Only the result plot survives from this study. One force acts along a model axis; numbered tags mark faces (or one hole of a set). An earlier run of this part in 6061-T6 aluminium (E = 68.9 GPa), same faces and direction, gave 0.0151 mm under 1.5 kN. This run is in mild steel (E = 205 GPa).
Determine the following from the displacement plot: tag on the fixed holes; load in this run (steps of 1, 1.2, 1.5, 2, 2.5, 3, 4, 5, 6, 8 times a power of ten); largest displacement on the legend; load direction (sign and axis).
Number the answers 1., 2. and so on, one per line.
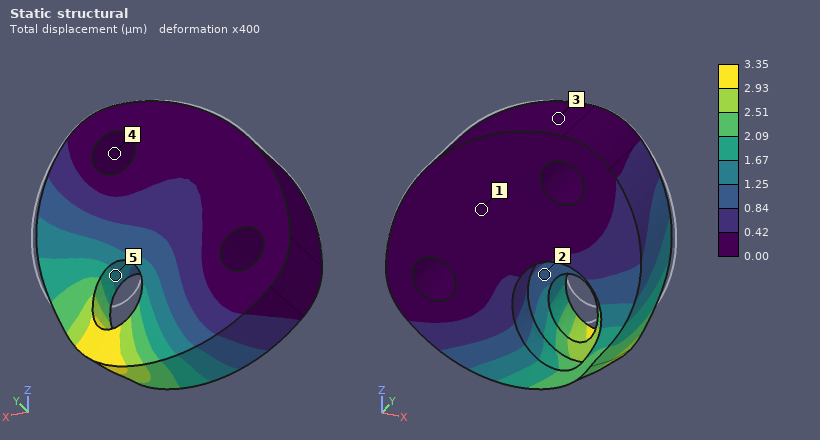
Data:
1. 4
2. 1 kN
3. 3.35 µm
4. -Z
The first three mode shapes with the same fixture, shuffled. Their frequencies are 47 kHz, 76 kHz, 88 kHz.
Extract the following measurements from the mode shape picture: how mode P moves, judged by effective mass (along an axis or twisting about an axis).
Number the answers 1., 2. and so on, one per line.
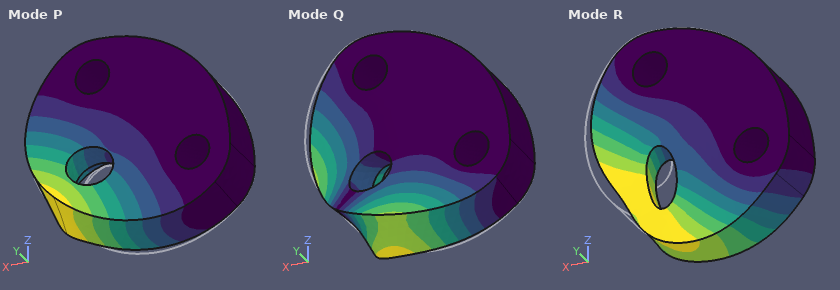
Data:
1. along Y
